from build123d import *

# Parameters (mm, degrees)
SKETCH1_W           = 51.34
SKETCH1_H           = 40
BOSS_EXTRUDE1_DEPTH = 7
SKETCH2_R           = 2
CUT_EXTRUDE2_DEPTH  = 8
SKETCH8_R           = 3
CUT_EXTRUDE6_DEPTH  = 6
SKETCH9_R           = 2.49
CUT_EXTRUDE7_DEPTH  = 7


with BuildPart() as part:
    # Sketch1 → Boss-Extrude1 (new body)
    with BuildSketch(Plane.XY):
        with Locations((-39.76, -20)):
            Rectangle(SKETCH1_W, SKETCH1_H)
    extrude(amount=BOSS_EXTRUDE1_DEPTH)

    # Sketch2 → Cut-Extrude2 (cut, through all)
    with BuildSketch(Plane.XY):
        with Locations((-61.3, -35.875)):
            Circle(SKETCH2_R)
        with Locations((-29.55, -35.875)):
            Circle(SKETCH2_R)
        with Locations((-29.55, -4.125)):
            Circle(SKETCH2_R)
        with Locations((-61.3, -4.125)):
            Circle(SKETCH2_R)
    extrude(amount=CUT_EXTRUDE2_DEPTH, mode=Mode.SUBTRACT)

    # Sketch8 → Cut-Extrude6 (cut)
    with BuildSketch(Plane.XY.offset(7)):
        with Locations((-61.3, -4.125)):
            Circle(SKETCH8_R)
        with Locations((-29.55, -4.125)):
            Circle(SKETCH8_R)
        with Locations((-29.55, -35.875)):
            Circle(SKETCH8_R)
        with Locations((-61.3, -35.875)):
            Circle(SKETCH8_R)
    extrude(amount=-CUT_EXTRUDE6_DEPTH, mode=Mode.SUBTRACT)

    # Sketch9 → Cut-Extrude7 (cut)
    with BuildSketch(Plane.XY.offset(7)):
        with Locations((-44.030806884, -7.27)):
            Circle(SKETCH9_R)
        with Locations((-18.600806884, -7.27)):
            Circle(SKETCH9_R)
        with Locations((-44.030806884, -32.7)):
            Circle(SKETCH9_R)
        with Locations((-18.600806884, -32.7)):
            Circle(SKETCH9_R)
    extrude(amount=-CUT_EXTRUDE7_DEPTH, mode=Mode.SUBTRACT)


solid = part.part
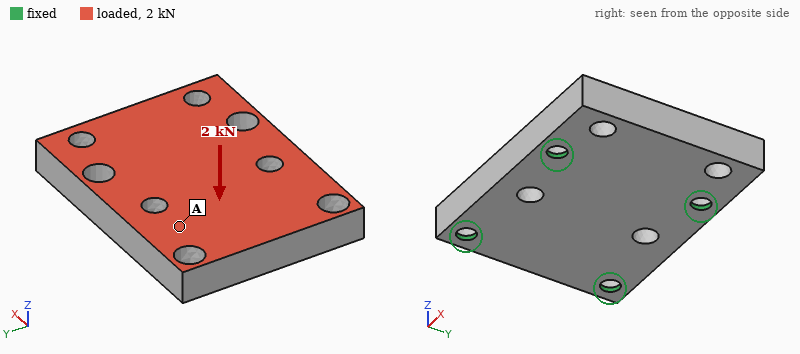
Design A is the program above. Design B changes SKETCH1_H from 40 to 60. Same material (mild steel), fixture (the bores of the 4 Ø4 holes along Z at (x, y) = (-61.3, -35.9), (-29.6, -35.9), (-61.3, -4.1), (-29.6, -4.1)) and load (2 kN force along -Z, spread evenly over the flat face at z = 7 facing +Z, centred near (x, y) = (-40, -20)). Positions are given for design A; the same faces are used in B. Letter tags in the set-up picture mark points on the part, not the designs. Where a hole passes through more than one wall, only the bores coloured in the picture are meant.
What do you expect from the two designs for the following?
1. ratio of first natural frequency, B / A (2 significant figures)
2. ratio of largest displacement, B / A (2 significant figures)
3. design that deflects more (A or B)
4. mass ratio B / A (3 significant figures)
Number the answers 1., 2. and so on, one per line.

1. 0.99
2. 0.63
3. A
4. 1.55
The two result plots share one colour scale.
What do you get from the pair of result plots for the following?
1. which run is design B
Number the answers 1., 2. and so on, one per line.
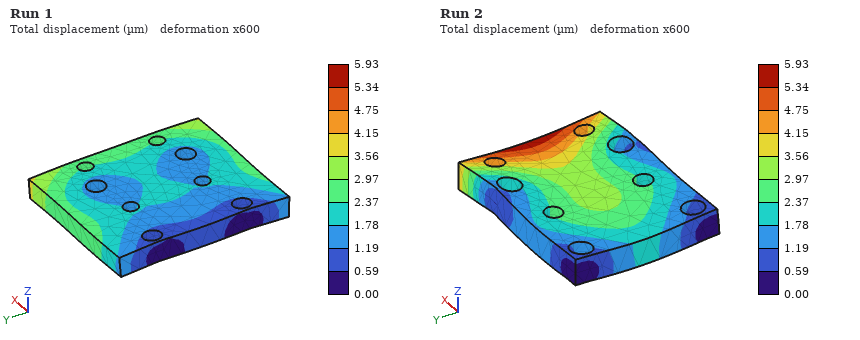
1. Run 1
